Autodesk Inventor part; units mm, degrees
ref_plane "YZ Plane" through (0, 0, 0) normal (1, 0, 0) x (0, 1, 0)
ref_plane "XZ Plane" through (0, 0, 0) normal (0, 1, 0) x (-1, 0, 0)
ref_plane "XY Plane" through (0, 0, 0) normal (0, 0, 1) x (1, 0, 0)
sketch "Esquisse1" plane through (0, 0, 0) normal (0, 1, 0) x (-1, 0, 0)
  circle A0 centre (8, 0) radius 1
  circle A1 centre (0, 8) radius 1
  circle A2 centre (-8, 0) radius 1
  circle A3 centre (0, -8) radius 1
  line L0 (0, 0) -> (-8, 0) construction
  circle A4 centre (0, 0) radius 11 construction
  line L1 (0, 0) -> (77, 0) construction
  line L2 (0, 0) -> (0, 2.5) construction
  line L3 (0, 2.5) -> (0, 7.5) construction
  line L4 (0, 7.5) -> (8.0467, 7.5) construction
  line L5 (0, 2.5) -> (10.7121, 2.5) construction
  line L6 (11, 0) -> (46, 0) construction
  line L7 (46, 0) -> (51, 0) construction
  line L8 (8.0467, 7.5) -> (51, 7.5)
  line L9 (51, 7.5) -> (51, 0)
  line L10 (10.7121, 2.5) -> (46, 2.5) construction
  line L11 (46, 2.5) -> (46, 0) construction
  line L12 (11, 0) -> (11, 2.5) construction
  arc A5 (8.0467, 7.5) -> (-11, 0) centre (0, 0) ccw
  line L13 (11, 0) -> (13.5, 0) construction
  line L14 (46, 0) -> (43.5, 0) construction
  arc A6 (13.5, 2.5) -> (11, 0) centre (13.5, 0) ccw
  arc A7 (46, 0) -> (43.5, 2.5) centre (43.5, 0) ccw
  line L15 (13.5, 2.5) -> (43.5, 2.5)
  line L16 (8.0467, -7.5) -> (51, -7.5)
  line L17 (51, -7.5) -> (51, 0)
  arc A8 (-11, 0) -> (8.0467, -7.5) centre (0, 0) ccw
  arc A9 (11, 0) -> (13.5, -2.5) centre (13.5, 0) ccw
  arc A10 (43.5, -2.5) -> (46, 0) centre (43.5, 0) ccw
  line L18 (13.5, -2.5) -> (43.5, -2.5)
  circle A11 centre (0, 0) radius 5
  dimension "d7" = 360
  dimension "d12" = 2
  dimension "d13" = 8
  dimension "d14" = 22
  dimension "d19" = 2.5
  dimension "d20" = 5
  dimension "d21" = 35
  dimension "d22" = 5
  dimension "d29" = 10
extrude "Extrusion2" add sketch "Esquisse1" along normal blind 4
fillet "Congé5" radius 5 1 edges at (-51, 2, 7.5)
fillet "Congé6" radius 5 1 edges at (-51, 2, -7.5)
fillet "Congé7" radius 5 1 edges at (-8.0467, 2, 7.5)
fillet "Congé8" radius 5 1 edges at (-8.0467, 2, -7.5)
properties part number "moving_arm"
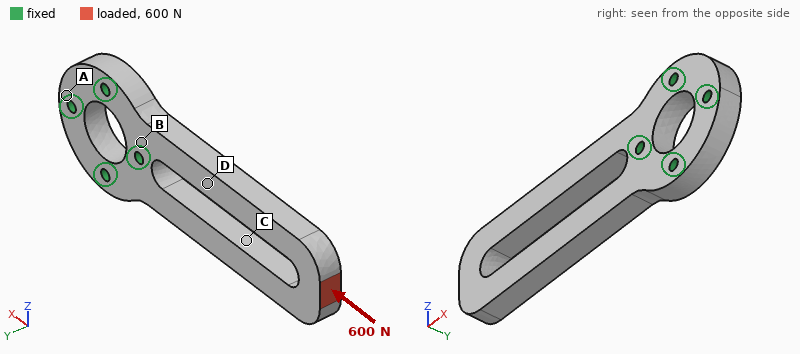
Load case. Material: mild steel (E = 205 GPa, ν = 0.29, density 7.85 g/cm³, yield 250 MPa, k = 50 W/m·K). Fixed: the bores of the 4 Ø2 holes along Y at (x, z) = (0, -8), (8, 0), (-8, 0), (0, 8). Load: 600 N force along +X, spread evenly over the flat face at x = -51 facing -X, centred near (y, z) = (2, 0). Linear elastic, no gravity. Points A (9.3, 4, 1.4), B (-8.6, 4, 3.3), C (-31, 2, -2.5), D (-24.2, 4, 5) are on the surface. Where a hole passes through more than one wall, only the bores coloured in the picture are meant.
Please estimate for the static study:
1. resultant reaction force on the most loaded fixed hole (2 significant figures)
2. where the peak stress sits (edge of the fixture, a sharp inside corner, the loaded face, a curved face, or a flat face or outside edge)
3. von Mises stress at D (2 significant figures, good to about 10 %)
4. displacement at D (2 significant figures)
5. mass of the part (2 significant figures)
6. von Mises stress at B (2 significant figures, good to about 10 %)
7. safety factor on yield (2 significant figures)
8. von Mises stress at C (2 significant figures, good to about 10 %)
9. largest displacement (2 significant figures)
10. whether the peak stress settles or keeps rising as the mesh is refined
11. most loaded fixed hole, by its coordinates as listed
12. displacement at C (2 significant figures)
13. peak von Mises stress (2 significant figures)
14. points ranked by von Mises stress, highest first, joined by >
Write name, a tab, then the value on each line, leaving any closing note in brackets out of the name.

resultant reaction force on the most loaded fixed hole	240 N
where the peak stress sits	a curved face
von Mises stress at D	15 MPa
displacement at D	2.3 µm
mass of the part	23 g
von Mises stress at B	8.2 MPa
safety factor on yield	3.3
von Mises stress at C	22 MPa
largest displacement	4.8 µm
whether the peak stress settles or keeps rising as the mesh is refined	settles
most loaded fixed hole, by its coordinates as listed	(-8, 0)
displacement at C	2.9 µm
peak von Mises stress	75 MPa
points ranked by von Mises stress, highest first, joined by >	C > D > B > A
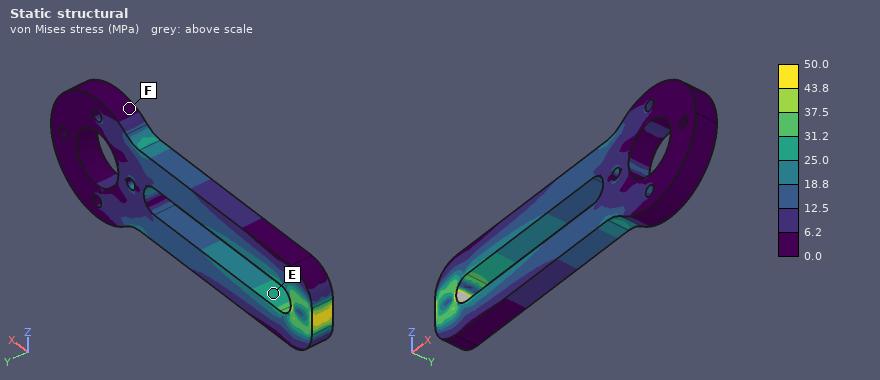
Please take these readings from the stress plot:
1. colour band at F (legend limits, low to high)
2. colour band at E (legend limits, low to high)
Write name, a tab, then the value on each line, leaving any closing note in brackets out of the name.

colour band at F	0.0 to 6.2 MPa
colour band at E	25.0 to 31.2 MPa
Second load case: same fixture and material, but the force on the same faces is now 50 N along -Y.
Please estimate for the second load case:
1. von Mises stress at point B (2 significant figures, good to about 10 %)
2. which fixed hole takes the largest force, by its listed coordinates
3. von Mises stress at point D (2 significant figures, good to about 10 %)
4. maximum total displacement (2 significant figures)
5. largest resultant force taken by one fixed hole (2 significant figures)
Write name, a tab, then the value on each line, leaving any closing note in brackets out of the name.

von Mises stress at point B	38 MPa
which fixed hole takes the largest force, by its listed coordinates	(-8, 0)
von Mises stress at point D	50 MPa
maximum total displacement	0.12 mm
largest resultant force taken by one fixed hole	160 N
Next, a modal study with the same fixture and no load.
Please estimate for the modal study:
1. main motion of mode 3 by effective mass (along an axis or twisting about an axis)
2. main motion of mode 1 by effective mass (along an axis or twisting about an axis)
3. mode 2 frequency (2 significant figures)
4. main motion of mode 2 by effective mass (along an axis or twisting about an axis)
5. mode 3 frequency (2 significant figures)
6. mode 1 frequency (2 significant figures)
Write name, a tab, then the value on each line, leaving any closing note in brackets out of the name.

main motion of mode 3 by effective mass	twisting about X
main motion of mode 1 by effective mass	along Y
mode 2 frequency	3500 Hz
main motion of mode 2 by effective mass	along Z
mode 3 frequency	6300 Hz
mode 1 frequency	1700 Hz
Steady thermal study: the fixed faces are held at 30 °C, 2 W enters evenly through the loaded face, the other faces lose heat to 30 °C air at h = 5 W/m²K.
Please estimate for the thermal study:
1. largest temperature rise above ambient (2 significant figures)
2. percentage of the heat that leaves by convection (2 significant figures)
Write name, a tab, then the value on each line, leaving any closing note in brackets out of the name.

largest temperature rise above ambient	43 K
percentage of the heat that leaves by convection	8.2 %
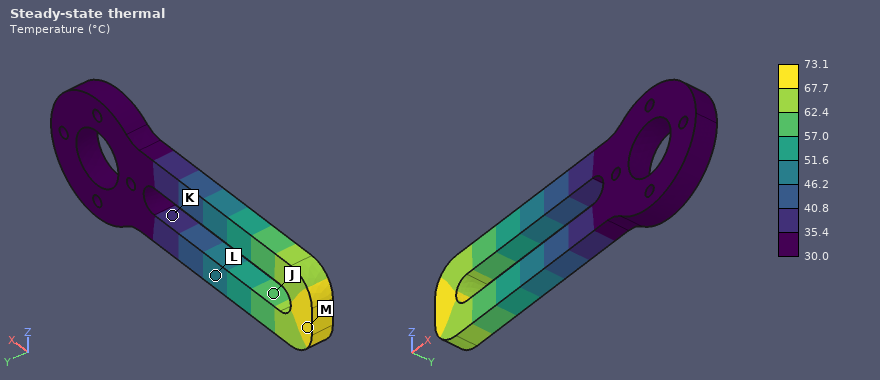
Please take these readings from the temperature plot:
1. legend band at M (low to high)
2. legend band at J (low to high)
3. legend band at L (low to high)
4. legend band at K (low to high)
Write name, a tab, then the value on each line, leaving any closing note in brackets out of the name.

legend band at M	67.7 to 73.1 °C
legend band at J	57.0 to 62.4 °C
legend band at L	46.2 to 51.6 °C
legend band at K	35.4 to 40.8 °C
